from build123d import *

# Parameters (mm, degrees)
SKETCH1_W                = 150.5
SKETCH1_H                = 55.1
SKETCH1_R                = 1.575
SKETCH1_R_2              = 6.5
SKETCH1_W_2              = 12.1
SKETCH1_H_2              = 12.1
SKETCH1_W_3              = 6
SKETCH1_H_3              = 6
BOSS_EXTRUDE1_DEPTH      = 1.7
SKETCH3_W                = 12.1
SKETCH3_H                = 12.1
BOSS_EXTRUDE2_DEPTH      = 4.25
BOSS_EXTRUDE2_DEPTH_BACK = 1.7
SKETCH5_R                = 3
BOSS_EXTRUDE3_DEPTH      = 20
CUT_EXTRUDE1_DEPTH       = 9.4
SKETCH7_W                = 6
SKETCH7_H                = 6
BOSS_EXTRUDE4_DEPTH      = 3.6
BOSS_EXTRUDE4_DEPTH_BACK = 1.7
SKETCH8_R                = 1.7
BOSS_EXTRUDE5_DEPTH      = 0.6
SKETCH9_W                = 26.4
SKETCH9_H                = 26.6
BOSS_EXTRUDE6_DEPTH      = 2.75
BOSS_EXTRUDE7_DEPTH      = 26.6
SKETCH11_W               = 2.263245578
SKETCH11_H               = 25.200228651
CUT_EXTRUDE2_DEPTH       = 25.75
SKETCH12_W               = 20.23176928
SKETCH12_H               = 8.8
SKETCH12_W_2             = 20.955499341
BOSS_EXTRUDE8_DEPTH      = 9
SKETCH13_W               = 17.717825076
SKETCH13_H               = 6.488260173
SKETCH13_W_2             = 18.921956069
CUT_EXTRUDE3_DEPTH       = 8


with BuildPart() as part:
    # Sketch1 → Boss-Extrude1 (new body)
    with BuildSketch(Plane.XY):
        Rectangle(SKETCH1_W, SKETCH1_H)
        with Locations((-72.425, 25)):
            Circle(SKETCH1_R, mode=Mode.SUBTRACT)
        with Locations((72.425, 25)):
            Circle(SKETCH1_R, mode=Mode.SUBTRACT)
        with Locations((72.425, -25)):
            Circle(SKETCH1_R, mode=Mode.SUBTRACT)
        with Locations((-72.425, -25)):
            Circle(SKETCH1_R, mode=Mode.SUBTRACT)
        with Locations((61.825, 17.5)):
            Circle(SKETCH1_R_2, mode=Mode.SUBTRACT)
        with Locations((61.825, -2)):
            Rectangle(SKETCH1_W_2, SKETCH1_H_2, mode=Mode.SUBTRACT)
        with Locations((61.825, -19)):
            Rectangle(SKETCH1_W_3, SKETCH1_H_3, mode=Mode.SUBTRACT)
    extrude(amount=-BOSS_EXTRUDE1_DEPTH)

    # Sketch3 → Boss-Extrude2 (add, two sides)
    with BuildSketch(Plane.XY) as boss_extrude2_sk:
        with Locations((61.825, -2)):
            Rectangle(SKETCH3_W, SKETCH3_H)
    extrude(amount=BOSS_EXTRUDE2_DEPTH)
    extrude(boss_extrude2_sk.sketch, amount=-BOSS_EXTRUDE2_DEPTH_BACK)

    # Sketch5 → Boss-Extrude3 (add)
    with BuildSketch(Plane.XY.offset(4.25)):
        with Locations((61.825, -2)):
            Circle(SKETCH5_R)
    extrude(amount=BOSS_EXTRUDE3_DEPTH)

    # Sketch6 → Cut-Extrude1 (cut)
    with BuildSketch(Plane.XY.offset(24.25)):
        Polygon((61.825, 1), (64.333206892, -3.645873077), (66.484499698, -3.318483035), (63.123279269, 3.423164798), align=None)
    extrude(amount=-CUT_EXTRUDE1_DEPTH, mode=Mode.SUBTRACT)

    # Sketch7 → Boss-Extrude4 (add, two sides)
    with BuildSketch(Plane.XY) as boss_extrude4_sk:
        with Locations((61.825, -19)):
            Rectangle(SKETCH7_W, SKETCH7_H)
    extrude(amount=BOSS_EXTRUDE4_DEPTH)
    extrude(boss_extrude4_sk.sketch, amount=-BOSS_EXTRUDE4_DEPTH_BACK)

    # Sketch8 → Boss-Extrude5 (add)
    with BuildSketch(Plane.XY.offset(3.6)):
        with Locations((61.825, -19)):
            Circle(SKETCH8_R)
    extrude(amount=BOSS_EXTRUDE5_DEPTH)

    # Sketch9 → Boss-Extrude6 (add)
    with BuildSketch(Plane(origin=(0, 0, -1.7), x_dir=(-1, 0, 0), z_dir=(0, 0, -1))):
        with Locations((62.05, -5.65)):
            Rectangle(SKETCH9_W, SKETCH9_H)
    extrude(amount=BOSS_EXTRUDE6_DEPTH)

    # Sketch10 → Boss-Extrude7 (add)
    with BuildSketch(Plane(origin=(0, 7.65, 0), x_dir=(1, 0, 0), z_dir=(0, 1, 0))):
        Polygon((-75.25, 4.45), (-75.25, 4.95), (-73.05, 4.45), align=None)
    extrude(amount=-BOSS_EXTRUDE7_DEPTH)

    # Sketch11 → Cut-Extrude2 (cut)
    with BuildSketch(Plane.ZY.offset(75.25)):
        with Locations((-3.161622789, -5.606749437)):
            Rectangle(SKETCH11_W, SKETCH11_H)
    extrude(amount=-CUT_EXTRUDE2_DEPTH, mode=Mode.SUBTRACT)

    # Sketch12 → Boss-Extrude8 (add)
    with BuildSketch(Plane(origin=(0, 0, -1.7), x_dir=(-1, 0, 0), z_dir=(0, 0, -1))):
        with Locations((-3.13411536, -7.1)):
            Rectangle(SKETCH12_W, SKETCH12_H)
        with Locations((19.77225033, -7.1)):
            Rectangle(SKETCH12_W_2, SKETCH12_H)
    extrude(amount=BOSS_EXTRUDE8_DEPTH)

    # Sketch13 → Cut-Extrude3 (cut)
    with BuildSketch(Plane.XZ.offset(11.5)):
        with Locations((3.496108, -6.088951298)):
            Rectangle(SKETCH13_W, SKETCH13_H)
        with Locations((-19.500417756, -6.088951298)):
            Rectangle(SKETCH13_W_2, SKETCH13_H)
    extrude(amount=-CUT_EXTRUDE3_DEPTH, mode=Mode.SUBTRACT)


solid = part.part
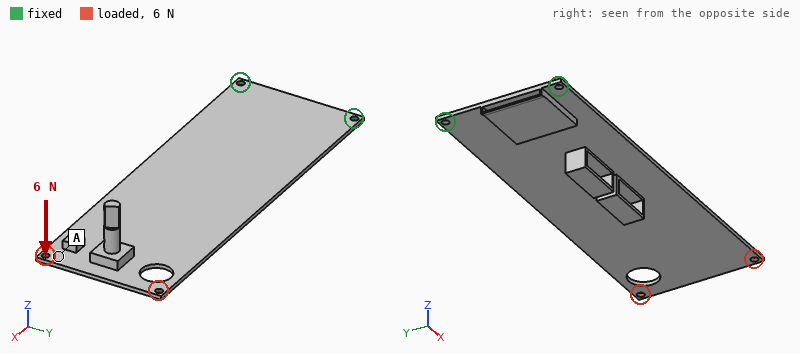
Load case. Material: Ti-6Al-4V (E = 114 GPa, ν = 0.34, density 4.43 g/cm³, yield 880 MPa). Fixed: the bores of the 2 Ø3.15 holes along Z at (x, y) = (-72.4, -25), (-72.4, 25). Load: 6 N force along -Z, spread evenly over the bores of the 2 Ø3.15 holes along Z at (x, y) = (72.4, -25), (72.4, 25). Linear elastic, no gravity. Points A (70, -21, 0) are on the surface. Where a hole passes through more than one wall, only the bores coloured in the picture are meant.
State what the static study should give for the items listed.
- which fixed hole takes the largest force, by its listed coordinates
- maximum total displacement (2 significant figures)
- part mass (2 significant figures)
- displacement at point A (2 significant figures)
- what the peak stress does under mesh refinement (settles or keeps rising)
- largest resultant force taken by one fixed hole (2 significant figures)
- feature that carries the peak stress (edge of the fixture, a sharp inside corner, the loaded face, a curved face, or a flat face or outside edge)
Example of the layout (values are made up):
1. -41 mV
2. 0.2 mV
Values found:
1. (-72.4, 25)
2. 2.0 mm
3. 75 g
4. 1.8 mm
5. keeps rising
6. 4.7 N
7. edge of the fixture
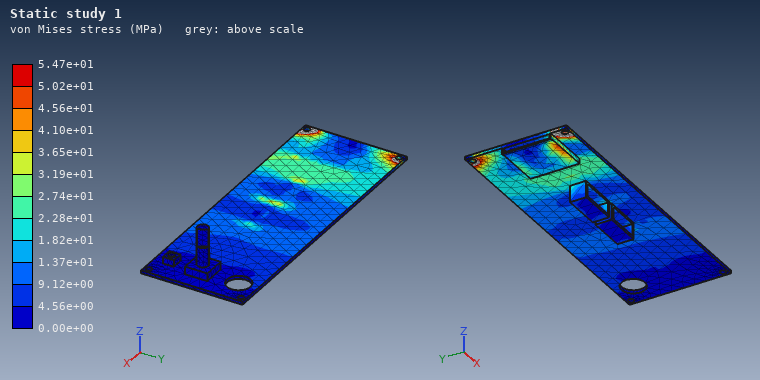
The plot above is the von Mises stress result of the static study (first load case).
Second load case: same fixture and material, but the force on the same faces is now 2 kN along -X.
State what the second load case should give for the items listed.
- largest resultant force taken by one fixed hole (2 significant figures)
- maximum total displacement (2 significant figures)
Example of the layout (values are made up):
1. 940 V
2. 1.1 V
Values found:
1. 1.1 kN
2. 0.20 mm
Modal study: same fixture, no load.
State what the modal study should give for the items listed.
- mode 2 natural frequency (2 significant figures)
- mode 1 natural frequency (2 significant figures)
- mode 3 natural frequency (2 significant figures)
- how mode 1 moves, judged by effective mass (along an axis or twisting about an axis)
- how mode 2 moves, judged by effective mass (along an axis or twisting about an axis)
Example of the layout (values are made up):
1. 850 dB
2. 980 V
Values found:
1. 390 Hz
2. 62 Hz
3. 420 Hz
4. along Z
5. along Z
